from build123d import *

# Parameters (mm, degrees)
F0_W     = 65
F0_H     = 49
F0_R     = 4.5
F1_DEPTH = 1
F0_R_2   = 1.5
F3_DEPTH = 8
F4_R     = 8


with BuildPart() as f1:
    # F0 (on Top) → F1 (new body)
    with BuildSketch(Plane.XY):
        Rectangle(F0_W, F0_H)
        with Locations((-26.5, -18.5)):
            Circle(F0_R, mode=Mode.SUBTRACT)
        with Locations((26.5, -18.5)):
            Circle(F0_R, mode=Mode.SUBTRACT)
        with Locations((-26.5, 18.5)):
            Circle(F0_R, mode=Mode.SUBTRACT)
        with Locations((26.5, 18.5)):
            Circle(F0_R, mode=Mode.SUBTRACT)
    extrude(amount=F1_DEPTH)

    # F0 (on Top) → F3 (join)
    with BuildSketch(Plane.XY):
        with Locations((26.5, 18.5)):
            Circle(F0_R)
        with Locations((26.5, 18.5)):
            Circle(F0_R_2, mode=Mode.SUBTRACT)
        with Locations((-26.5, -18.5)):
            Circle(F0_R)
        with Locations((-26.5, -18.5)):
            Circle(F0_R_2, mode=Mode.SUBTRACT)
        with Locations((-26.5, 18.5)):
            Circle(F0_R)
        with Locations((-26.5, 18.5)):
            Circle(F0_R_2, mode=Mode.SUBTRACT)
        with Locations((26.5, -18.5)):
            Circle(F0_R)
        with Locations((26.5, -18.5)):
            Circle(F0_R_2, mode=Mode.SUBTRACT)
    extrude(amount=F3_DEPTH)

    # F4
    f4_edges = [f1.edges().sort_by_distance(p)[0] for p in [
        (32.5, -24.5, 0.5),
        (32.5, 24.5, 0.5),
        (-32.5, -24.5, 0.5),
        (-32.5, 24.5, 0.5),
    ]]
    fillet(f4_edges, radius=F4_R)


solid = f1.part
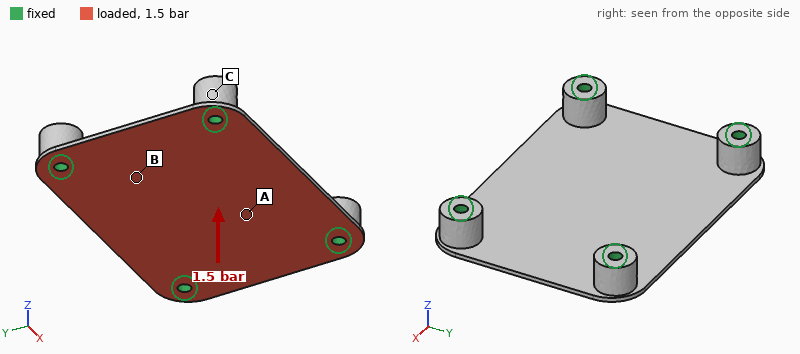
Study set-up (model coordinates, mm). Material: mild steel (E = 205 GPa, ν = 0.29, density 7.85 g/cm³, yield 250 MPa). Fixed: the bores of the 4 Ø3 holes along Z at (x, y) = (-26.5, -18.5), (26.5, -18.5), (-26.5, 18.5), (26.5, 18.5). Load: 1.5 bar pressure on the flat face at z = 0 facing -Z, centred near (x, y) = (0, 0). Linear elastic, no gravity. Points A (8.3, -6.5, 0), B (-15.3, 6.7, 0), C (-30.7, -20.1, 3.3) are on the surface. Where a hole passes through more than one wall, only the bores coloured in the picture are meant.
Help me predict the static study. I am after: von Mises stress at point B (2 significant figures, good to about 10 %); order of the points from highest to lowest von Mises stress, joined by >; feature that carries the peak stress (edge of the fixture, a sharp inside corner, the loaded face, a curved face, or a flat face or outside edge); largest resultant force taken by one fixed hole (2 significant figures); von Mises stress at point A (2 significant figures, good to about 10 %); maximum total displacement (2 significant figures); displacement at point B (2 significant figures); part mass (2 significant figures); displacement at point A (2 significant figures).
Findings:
37 MPa
A > B > C
the loaded face
130 N
59 MPa
0.16 mm
0.079 mm
37 g
0.13 mm
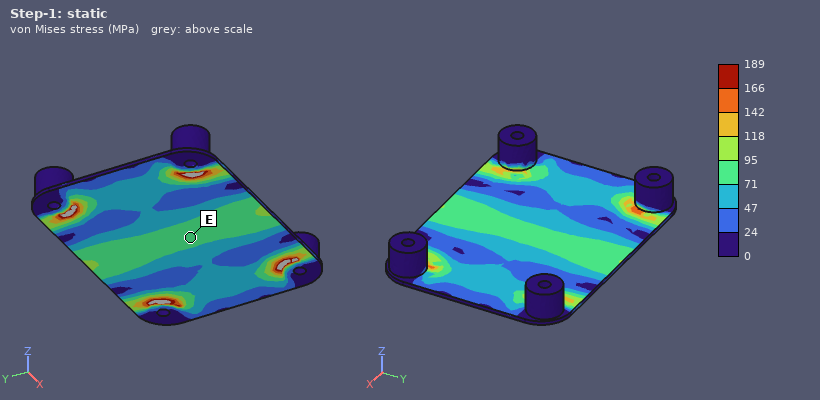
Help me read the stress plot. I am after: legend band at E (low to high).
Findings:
71 to 95 MPa
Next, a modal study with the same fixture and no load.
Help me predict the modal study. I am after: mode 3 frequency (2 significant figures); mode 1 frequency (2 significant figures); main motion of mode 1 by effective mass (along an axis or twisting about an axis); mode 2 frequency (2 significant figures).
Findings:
4100 Hz
2100 Hz
along Z
2900 Hz
